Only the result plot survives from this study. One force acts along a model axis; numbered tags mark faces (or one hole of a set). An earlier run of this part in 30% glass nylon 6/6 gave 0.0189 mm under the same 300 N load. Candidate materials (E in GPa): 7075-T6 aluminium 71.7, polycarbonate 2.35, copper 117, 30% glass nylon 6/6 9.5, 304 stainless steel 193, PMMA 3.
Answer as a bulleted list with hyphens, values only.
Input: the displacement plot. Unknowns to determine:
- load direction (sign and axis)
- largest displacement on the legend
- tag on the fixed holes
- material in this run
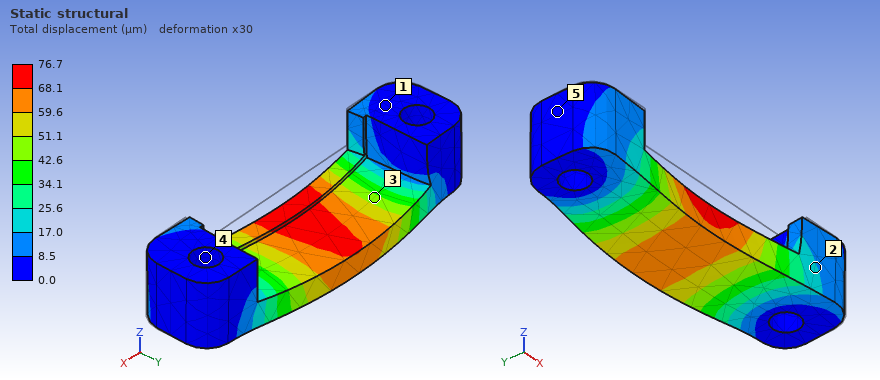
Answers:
- +Y
- 76.7 µm
- 4
- polycarbonate
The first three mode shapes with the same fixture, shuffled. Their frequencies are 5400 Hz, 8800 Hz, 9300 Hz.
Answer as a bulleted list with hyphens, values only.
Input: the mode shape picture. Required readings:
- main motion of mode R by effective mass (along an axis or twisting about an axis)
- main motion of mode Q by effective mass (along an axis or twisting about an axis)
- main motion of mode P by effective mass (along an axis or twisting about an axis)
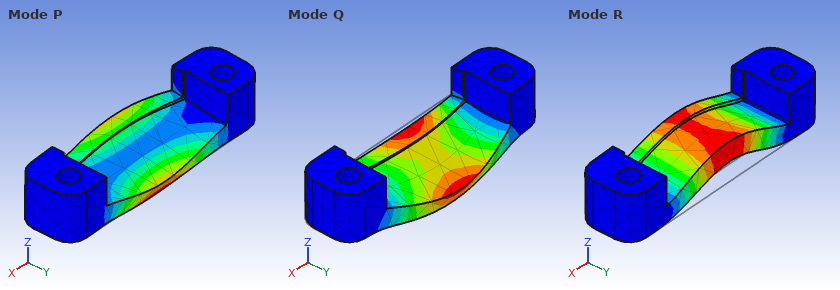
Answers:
- along Z
- along Y
- along Y
